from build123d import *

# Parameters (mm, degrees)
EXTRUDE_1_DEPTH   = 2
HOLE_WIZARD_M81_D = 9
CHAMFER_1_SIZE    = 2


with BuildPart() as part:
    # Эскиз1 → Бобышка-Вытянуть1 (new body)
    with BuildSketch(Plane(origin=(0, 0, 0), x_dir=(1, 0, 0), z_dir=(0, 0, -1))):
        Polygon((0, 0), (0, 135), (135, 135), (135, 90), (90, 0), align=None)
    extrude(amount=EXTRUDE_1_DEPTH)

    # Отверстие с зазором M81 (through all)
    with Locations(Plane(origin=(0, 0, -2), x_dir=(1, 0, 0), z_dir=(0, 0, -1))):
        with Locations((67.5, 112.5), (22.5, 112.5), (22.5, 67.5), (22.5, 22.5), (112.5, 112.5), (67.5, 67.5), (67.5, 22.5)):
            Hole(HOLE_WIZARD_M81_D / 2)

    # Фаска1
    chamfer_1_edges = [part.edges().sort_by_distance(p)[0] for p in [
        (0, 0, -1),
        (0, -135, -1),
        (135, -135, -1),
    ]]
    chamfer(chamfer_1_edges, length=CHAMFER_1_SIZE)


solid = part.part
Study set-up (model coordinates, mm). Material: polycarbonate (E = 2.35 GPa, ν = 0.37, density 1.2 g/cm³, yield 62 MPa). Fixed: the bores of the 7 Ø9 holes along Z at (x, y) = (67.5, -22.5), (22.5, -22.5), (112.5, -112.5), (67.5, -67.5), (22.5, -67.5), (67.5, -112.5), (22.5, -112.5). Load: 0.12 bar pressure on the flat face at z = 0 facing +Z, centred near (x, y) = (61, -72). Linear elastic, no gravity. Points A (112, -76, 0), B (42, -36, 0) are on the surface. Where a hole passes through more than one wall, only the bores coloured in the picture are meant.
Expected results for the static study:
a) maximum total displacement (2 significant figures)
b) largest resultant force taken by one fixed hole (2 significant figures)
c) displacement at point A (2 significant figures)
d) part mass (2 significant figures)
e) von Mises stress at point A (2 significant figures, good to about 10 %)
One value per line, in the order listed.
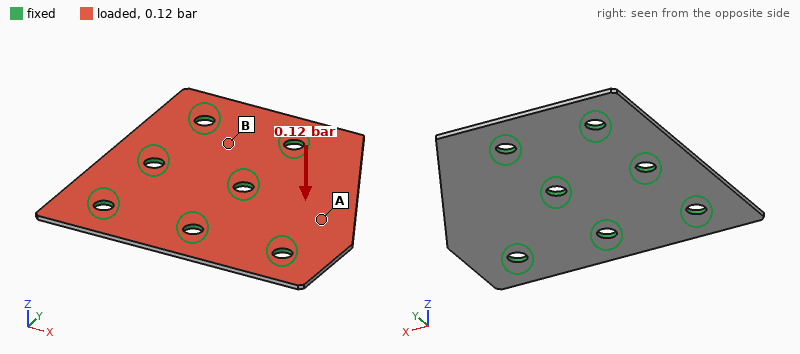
2.1 mm
34 N
1.1 mm
38 g
3.5 MPa
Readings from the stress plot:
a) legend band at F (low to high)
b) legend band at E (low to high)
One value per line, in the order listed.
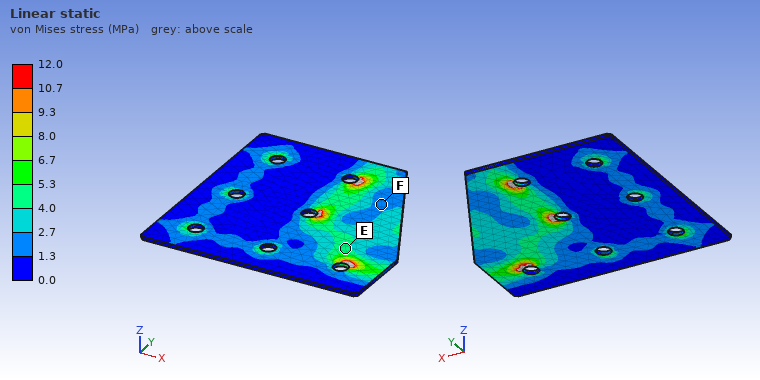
1.3 to 2.7 MPa
4.0 to 5.3 MPa
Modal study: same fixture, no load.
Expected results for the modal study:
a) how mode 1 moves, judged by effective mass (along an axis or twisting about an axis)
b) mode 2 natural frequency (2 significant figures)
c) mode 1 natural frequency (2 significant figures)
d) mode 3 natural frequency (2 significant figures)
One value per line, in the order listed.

along Z
630 Hz
330 Hz
860 Hz
